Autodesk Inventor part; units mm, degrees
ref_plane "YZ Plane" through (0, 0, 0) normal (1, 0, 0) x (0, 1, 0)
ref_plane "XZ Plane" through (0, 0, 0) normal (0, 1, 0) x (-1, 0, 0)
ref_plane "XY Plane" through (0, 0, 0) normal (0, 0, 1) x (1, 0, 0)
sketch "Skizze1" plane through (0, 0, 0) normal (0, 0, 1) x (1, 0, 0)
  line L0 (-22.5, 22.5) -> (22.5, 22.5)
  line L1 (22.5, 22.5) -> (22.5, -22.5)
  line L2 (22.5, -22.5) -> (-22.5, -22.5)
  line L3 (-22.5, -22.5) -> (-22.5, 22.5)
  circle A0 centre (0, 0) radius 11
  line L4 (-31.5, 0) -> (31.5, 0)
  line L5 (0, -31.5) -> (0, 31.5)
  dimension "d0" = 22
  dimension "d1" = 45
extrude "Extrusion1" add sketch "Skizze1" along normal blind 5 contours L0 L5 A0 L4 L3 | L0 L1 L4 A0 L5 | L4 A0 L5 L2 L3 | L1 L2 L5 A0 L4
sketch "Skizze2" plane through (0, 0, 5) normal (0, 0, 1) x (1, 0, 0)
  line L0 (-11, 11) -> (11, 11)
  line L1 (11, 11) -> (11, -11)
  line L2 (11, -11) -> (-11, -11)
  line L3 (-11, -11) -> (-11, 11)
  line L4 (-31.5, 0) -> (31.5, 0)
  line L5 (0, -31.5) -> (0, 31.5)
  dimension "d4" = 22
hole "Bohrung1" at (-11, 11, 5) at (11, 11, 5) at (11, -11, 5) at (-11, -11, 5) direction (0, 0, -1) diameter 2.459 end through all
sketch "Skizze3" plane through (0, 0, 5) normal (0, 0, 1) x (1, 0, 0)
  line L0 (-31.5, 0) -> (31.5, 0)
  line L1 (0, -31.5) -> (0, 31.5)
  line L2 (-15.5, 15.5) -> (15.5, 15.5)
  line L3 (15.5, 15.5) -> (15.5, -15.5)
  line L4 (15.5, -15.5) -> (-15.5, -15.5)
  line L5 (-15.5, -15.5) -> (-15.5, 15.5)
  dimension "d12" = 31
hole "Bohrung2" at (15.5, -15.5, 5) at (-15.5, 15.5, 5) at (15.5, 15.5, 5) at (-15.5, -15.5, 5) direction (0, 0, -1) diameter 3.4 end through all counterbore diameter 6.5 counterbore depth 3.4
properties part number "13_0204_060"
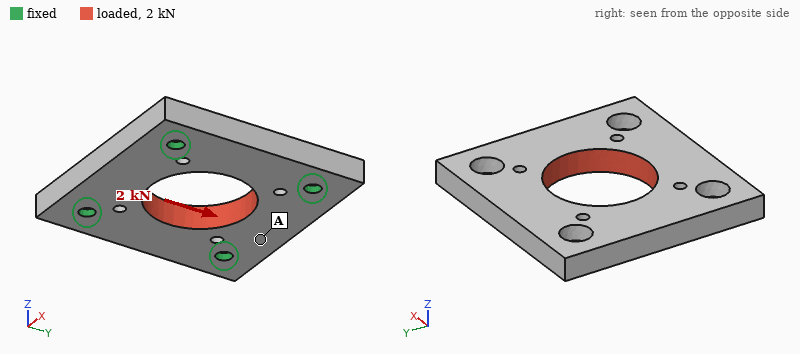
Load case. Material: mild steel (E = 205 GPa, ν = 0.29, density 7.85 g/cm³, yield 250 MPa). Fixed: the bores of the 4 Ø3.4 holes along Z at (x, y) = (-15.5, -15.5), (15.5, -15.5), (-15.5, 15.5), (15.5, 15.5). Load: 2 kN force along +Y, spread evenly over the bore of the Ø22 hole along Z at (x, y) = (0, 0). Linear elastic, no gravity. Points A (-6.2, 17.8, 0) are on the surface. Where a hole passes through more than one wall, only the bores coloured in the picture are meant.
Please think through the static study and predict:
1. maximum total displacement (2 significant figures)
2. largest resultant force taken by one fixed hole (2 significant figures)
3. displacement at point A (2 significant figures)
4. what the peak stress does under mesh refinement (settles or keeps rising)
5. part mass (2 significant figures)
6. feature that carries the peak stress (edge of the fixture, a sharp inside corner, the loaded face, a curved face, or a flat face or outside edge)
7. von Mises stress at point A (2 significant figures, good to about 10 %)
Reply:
1.9 µm
510 N
1.0 µm
keeps rising
60 g
edge of the fixture
6.4 MPa
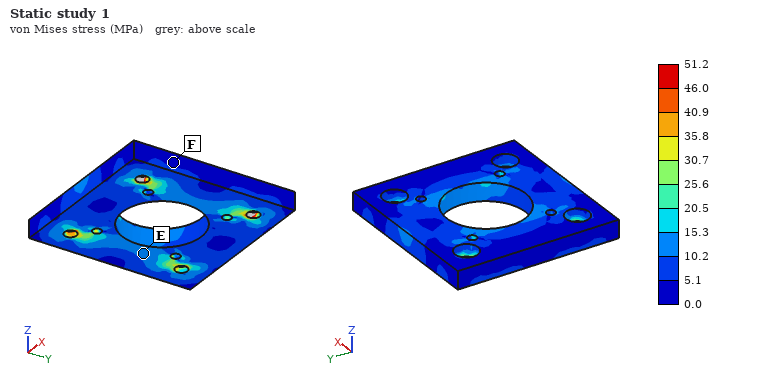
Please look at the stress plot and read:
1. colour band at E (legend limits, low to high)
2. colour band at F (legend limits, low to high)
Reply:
10.2 to 15.3 MPa
0.0 to 5.1 MPa
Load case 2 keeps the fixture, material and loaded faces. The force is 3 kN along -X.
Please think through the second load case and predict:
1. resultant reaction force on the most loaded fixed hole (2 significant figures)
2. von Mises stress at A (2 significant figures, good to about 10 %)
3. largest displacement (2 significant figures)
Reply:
760 N
14 MPa
2.8 µm
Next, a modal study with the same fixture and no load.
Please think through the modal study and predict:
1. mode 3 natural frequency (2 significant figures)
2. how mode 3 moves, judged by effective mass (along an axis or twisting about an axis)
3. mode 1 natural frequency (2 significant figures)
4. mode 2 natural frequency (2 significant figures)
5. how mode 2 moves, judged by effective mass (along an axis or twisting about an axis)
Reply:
18 kHz
twisting about X
15 kHz
16 kHz
along Z
